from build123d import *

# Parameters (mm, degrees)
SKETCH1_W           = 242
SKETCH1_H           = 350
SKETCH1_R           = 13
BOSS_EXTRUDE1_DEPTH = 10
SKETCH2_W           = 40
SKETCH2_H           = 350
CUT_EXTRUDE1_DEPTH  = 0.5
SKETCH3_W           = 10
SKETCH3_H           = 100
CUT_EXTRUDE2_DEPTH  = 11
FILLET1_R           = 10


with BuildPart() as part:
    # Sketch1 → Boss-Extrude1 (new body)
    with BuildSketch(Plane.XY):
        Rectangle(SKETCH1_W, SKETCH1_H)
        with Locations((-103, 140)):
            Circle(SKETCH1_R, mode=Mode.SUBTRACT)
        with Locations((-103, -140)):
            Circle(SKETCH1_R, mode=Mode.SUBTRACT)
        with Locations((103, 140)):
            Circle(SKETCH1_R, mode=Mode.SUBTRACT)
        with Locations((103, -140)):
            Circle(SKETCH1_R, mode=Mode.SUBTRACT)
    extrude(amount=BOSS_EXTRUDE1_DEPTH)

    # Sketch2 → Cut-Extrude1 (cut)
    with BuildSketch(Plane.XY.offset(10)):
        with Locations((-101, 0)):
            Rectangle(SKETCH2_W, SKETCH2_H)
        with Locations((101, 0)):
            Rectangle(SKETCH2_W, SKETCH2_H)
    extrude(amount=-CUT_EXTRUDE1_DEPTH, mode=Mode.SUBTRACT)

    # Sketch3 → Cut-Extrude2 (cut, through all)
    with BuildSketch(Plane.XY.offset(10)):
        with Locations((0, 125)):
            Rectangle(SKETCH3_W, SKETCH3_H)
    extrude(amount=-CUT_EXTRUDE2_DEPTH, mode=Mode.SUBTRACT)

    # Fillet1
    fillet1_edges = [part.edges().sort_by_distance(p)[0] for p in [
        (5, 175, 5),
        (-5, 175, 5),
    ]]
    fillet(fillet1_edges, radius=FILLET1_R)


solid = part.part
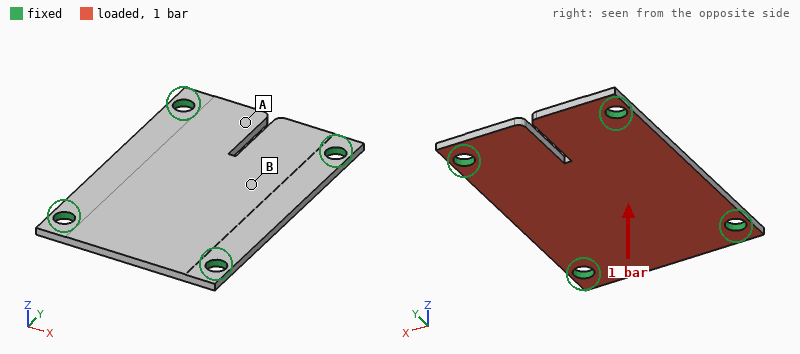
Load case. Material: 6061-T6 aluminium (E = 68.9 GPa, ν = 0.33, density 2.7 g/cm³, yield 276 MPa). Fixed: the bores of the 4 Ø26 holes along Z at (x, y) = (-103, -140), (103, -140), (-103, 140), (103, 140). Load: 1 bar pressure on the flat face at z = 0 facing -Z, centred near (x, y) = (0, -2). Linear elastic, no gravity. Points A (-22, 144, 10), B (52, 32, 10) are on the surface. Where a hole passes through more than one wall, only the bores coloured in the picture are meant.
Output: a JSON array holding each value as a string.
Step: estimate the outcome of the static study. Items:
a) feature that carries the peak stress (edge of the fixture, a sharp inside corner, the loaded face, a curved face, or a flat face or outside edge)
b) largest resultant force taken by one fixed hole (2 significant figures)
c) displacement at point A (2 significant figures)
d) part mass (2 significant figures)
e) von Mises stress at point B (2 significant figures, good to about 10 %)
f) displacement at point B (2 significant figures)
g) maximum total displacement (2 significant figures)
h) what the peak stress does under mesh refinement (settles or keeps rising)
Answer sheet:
["edge of the fixture", "2.1 kN", "0.12 mm", "2.2 kg", "17 MPa", "0.33 mm", "0.38 mm", "keeps rising"]
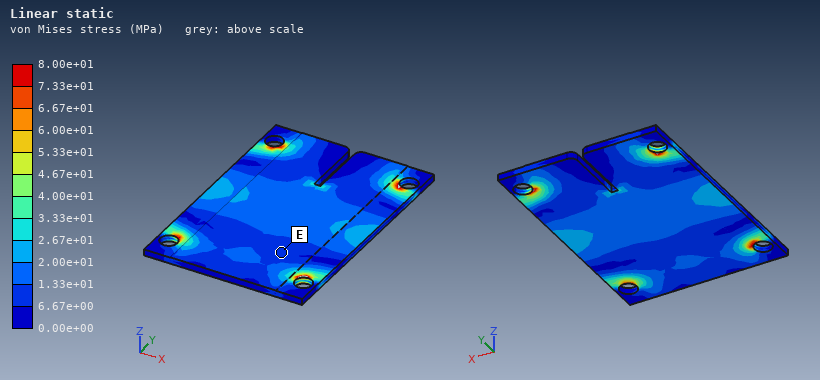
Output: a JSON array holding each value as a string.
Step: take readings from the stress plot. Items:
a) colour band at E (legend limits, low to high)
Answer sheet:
["6.67e+00 to 1.33e+01 MPa"]
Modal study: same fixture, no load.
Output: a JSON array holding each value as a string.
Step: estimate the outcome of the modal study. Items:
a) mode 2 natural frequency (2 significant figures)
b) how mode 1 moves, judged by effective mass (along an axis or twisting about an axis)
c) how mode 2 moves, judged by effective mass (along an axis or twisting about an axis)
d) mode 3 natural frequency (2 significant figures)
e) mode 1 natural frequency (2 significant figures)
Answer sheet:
["880 Hz", "along Z", "twisting about Y", "1100 Hz", "590 Hz"]
